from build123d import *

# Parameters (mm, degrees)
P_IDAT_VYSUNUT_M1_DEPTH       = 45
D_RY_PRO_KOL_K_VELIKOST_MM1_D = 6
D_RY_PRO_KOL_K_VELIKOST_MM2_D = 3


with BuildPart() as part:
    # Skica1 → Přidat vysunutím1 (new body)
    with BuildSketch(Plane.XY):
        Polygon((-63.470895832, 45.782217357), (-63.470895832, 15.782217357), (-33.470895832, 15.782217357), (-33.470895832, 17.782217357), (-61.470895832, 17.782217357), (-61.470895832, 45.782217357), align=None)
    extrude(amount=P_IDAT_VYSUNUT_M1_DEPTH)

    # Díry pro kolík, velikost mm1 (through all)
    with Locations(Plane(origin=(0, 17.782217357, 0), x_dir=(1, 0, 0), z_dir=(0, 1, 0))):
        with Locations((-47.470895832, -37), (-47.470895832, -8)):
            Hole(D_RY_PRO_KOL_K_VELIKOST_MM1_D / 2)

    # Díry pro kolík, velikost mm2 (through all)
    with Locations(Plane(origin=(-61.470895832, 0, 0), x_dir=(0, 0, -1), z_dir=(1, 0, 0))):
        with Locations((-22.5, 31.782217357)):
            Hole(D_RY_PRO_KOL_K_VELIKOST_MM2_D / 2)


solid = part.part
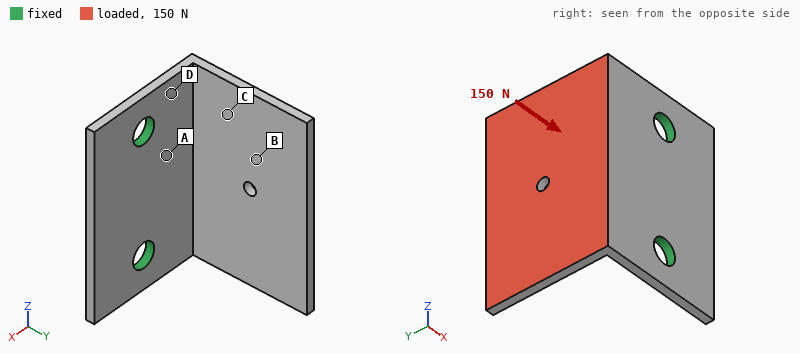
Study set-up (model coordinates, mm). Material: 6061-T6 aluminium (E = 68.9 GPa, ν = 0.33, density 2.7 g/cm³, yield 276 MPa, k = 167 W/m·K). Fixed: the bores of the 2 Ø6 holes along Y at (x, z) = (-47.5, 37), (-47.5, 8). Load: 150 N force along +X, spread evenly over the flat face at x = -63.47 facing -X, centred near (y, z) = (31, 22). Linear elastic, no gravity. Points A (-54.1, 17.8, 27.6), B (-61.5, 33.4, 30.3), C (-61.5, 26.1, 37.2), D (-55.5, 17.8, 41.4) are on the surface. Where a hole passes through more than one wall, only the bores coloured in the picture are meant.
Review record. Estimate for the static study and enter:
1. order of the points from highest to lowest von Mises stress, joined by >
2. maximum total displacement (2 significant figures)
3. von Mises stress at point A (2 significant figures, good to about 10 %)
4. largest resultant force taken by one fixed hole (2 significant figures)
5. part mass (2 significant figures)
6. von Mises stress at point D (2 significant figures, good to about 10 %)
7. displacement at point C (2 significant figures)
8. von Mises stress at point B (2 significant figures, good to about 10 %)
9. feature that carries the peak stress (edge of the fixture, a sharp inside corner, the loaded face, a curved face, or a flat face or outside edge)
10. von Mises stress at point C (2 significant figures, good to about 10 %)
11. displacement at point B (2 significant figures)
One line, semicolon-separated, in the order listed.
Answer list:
D > A > C > B; 0.56 mm; 55 MPa; 77 N; 14 g; 69 MPa; 0.16 mm; 13 MPa; a flat face or outside edge; 29 MPa; 0.30 mm
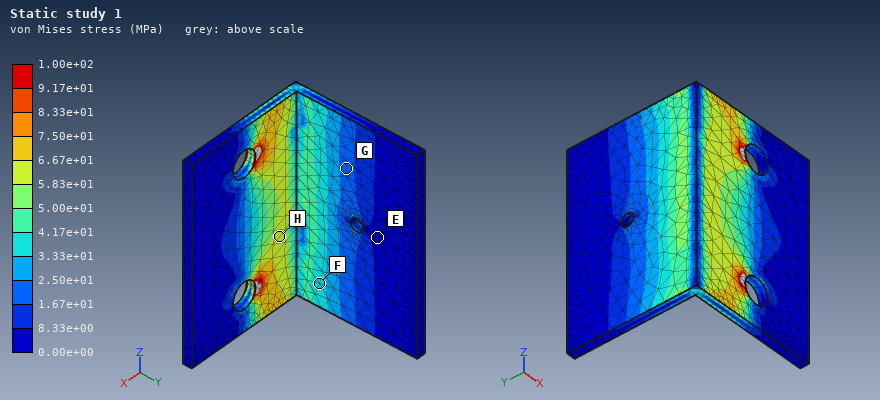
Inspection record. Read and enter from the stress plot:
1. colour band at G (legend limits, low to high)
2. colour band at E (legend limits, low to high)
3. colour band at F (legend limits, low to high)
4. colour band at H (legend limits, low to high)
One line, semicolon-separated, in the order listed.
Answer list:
1.67e+01 to 2.50e+01 MPa; 0.00e+00 to 8.33e+00 MPa; 3.33e+01 to 4.17e+01 MPa; 5.83e+01 to 6.67e+01 MPa
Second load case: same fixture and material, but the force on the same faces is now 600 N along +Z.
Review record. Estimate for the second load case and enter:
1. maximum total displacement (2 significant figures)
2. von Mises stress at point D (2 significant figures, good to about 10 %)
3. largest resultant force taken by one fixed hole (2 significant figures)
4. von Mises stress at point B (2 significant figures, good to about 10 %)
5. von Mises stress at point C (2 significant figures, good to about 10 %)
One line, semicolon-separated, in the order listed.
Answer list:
0.32 mm; 69 MPa; 490 N; 18 MPa; 40 MPa
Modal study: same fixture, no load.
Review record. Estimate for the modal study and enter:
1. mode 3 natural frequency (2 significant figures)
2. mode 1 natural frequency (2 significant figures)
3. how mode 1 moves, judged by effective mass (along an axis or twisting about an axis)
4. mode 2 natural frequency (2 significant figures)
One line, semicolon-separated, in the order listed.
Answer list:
3700 Hz; 1200 Hz; along X; 2400 Hz
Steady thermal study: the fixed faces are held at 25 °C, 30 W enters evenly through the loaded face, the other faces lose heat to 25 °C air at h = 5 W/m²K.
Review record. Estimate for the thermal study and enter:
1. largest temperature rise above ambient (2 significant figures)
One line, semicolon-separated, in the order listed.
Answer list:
57 K
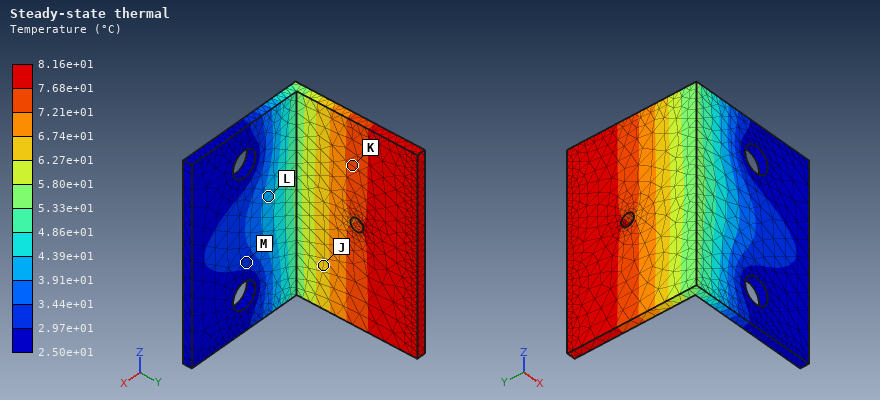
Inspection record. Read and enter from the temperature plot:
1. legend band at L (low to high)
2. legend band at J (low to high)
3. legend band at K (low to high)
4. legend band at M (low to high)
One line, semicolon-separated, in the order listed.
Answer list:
3.91e+01 to 4.39e+01 °C; 6.27e+01 to 6.74e+01 °C; 7.21e+01 to 7.68e+01 °C; 2.97e+01 to 3.44e+01 °C
